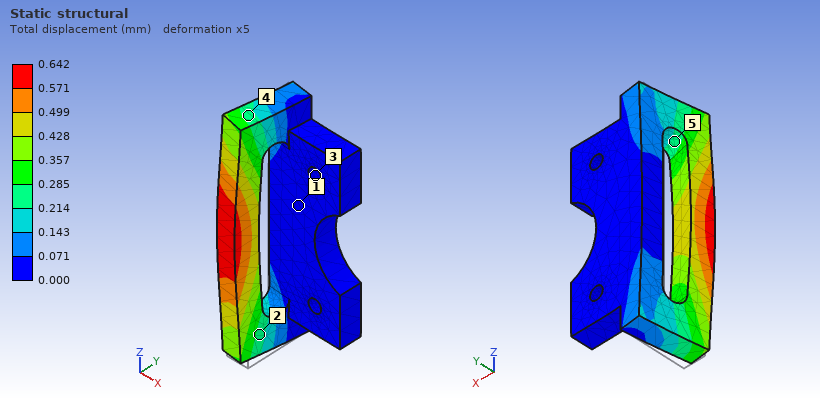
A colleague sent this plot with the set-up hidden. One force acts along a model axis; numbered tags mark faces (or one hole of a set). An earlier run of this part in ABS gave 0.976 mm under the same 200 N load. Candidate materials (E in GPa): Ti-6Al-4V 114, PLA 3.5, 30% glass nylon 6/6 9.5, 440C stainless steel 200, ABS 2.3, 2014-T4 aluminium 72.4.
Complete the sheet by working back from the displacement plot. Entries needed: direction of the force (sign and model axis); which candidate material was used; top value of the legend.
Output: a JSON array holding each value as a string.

["-X", "PLA", "0.642 mm"]
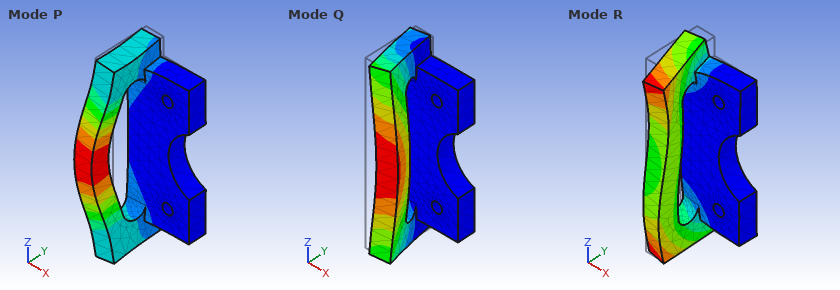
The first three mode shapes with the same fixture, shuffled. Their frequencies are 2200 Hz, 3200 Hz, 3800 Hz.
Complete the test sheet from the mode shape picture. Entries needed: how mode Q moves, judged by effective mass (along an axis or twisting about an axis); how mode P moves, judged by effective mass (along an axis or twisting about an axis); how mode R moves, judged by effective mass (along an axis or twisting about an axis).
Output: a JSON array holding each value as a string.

["along X", "along Y", "along Z"]
